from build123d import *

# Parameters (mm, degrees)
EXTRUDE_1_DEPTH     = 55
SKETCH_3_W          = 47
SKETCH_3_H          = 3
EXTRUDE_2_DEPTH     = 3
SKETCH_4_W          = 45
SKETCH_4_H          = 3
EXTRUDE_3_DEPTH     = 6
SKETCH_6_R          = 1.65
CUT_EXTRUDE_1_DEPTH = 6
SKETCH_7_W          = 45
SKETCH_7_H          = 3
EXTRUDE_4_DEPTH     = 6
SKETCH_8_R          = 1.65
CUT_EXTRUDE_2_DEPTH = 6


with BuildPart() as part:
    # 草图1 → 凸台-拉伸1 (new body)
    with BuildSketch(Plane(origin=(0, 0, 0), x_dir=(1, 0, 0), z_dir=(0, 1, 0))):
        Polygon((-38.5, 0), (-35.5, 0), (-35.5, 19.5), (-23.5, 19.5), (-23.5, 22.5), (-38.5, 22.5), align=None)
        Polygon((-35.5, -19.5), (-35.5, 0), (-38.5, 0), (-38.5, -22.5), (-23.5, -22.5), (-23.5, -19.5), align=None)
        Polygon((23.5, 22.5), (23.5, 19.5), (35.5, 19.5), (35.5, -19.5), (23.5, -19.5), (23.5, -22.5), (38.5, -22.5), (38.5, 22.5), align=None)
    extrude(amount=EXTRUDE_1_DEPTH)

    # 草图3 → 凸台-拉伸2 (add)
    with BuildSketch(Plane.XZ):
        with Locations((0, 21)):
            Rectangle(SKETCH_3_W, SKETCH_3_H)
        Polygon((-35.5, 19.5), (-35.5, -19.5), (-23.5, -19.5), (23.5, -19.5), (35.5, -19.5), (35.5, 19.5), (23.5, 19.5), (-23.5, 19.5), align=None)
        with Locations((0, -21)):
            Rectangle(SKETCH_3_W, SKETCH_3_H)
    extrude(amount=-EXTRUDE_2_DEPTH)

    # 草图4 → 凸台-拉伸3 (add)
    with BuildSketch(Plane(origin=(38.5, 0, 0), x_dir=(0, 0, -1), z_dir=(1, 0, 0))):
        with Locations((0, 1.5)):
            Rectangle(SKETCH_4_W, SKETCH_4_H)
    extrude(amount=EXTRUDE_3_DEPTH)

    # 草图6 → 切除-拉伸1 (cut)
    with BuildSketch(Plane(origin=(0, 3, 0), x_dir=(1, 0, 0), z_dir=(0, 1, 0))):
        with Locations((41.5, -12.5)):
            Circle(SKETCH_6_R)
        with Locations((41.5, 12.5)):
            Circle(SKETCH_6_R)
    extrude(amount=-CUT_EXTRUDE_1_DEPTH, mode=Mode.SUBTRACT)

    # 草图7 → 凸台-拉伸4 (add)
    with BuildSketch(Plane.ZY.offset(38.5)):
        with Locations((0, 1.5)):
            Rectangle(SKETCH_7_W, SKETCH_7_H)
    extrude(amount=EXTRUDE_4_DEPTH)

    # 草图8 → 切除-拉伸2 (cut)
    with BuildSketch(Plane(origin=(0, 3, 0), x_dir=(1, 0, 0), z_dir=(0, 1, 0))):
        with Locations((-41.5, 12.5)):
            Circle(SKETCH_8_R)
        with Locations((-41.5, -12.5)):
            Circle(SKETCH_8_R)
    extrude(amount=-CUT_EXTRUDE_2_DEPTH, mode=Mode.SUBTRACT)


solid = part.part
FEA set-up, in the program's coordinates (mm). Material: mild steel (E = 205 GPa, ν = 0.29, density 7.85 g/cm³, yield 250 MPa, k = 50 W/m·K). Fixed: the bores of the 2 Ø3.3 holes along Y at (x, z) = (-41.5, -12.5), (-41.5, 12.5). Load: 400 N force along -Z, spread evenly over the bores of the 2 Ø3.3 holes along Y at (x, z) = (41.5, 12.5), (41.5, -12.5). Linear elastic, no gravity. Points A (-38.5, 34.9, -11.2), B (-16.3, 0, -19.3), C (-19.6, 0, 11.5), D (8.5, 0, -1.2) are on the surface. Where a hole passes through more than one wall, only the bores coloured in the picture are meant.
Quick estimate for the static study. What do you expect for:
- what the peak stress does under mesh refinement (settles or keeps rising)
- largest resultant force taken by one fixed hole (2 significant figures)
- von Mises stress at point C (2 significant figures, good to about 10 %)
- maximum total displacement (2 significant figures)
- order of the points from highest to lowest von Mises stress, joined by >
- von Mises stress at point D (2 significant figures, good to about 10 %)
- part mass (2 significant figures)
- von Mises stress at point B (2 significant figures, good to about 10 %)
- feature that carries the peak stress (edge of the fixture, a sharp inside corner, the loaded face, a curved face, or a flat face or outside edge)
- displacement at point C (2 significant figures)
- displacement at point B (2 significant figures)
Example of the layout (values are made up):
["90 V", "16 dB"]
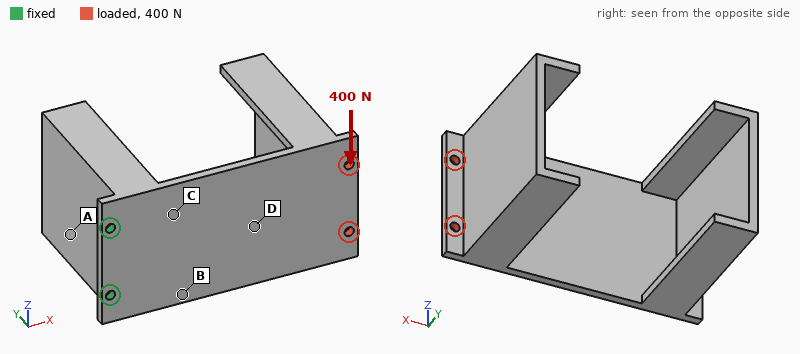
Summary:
["keeps rising", "1.2 kN", "13 MPa", "29 µm", "B > C > D > A", "7.8 MPa", "260 g", "18 MPa", "edge of the fixture", "5.2 µm", "7.2 µm"]
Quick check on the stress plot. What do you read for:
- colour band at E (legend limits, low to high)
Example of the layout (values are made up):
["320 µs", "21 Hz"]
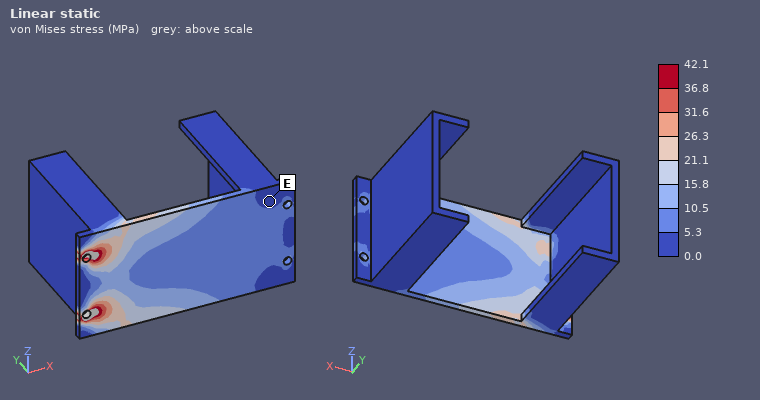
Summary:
["0.0 to 5.3 MPa"]
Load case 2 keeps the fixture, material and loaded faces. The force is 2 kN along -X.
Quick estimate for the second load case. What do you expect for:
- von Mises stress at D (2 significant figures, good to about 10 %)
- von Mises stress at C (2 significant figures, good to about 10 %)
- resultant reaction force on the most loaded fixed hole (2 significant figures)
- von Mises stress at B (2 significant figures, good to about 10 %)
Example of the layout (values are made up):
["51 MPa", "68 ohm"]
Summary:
["15 MPa", "15 MPa", "1.0 kN", "15 MPa"]
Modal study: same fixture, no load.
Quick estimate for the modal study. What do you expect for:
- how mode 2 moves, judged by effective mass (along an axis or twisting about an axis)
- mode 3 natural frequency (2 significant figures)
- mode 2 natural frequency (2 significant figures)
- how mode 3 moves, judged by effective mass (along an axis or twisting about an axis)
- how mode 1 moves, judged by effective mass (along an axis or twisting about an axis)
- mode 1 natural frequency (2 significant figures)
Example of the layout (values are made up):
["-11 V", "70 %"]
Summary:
["along Z", "640 Hz", "410 Hz", "along Y", "along Y", "170 Hz"]
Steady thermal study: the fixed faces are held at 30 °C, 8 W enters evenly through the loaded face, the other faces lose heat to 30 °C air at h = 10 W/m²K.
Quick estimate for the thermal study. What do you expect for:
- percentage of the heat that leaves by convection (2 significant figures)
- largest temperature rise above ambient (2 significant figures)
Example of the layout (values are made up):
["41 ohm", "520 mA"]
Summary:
["62 %", "56 K"]
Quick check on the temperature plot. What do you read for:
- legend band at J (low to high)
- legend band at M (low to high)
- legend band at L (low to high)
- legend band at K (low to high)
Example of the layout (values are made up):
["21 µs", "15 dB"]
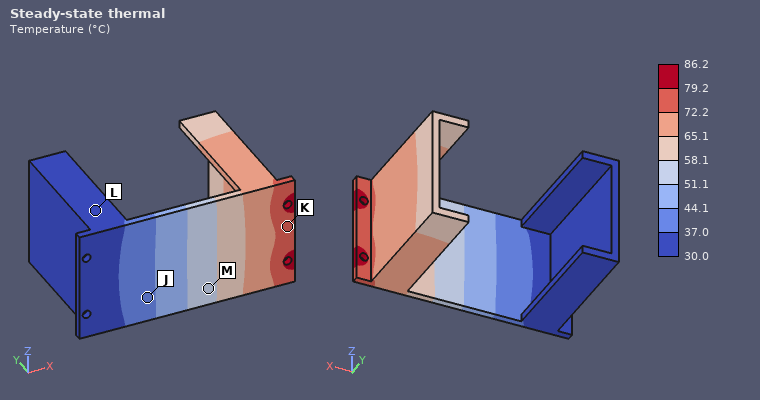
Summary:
["37.0 to 44.1 °C", "51.1 to 58.1 °C", "30.0 to 37.0 °C", "72.2 to 79.2 °C"]
